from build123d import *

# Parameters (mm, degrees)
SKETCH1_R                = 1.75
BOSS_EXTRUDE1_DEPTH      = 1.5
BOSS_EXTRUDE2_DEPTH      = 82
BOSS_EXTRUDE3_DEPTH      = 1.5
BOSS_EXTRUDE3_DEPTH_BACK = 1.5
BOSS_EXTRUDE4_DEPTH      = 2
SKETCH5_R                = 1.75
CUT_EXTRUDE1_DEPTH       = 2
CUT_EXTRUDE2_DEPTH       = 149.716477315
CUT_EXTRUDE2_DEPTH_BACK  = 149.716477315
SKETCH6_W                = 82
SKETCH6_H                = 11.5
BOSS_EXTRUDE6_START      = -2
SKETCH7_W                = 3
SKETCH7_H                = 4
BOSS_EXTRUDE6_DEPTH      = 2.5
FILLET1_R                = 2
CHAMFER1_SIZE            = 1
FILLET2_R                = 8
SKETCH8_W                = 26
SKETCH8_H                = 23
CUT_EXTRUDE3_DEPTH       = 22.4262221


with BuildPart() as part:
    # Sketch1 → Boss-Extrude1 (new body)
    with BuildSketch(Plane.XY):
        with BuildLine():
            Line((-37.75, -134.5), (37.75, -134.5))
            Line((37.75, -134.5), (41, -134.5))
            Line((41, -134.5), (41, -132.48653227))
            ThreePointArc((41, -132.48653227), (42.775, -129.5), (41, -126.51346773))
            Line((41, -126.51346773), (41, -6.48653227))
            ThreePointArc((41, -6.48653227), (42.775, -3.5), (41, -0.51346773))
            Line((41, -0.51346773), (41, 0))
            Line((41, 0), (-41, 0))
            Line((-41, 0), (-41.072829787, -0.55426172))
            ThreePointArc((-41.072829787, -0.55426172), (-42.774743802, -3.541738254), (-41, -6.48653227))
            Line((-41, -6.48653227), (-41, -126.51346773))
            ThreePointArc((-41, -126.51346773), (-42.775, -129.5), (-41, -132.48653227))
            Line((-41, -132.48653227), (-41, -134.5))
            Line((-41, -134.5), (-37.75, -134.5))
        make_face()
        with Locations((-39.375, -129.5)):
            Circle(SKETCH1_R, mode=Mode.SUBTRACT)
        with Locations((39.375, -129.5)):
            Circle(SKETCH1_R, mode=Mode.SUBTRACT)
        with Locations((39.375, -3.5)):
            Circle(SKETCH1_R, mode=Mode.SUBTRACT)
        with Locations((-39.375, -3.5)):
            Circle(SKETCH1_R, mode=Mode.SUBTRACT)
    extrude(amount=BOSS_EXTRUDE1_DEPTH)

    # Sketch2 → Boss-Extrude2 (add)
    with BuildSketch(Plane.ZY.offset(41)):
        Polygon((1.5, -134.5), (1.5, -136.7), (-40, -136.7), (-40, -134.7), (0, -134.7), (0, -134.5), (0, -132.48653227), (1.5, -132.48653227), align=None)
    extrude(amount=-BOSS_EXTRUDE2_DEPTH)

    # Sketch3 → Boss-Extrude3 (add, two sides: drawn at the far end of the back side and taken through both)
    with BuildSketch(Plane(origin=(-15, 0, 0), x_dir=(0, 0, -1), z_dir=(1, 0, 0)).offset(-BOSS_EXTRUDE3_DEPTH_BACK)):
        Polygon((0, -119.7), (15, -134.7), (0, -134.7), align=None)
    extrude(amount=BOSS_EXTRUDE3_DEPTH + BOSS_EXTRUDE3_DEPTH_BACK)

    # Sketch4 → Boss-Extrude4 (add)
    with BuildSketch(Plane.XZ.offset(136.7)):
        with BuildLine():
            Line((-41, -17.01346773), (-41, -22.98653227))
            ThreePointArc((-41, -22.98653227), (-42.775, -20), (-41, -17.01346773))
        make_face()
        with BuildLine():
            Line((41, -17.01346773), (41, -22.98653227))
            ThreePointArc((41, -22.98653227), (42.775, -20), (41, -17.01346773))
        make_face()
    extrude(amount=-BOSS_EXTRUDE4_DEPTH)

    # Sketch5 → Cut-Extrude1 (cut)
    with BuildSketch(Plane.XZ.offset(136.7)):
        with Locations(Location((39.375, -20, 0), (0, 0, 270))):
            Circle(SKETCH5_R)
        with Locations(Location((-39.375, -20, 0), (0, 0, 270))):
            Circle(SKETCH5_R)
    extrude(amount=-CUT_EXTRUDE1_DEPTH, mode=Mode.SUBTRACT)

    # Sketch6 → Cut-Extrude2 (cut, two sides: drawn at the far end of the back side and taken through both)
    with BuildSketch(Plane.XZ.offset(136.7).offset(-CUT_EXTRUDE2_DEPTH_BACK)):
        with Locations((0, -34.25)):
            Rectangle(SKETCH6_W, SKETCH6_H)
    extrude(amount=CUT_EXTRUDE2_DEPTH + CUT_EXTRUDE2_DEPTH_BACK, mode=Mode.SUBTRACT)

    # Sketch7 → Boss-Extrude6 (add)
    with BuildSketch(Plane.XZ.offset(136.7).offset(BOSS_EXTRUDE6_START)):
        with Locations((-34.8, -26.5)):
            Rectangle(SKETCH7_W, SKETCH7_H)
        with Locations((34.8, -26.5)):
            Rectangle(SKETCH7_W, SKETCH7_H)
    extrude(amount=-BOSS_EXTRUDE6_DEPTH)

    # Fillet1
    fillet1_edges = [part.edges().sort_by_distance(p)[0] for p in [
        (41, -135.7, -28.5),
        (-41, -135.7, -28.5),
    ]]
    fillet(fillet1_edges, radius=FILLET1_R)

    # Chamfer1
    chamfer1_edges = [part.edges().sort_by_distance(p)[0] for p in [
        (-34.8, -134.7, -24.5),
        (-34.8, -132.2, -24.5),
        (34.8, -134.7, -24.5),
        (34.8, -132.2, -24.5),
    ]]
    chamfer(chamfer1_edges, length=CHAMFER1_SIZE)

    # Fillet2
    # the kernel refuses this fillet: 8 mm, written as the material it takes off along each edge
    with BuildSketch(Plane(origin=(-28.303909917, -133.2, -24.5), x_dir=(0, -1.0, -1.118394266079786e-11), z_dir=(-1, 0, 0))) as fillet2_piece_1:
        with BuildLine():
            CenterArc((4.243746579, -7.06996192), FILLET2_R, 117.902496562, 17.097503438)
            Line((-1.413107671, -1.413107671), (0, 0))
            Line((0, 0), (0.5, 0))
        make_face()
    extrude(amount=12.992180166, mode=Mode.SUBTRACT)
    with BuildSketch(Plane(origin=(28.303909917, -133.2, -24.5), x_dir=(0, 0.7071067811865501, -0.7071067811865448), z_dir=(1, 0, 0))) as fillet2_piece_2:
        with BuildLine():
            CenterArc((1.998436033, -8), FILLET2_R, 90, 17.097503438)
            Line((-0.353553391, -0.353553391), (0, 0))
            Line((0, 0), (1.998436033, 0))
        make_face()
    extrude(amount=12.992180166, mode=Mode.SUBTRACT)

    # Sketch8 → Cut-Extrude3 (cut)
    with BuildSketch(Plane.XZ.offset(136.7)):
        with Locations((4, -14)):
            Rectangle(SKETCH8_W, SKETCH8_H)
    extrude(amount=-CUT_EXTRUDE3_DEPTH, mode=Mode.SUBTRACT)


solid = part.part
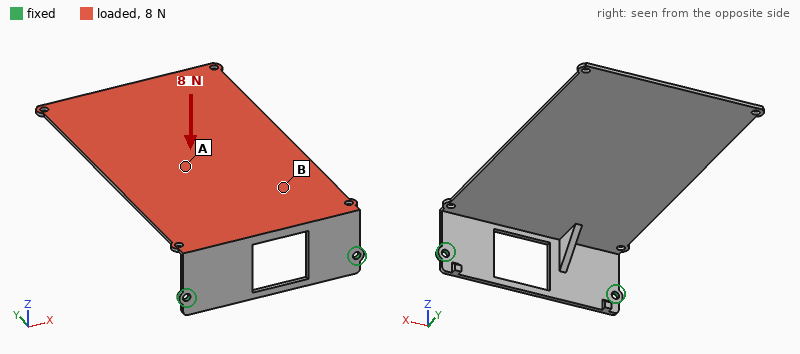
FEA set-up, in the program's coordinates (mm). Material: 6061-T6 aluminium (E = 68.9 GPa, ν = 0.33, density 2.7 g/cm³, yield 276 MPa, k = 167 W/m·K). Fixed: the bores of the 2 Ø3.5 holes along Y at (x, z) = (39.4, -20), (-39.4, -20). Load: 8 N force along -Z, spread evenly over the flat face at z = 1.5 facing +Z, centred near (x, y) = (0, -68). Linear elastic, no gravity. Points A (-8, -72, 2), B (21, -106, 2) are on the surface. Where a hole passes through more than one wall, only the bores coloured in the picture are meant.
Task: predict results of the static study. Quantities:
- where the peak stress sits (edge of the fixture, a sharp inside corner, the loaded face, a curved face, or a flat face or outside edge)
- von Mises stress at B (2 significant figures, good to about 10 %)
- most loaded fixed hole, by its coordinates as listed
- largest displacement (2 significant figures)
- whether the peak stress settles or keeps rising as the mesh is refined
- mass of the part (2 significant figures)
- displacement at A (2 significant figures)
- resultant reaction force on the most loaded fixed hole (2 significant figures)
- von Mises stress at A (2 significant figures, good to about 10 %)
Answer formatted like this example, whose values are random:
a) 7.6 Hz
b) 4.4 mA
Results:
a) edge of the fixture
b) 8.8 MPa
c) (-39.4, -20)
d) 1.8 mm
e) keeps rising
f) 56 g
g) 0.61 mm
h) 6.0 N
i) 4.4 MPa
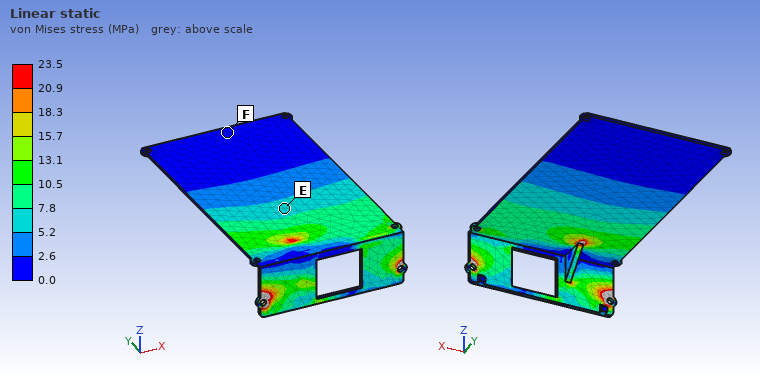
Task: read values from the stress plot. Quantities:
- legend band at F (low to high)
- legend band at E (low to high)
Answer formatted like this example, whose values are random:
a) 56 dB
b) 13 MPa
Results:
a) 0.0 to 2.6 MPa
b) 5.2 to 7.8 MPa
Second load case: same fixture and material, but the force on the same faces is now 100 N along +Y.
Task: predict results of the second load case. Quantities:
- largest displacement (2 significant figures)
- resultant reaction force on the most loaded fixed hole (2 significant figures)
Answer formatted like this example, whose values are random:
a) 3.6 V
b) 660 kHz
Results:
a) 1.7 mm
b) 51 N
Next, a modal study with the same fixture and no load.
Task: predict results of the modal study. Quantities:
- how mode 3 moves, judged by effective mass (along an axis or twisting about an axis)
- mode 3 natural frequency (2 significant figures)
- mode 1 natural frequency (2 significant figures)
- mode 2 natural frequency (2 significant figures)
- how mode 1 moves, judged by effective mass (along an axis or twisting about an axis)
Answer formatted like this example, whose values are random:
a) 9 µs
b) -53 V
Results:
a) along X
b) 320 Hz
c) 63 Hz
d) 230 Hz
e) along Z
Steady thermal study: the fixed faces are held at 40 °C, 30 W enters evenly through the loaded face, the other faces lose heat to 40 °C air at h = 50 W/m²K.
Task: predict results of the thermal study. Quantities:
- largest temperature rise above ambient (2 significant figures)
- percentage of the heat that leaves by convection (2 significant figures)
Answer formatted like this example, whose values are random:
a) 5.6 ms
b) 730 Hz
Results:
a) 41 K
b) 72 %
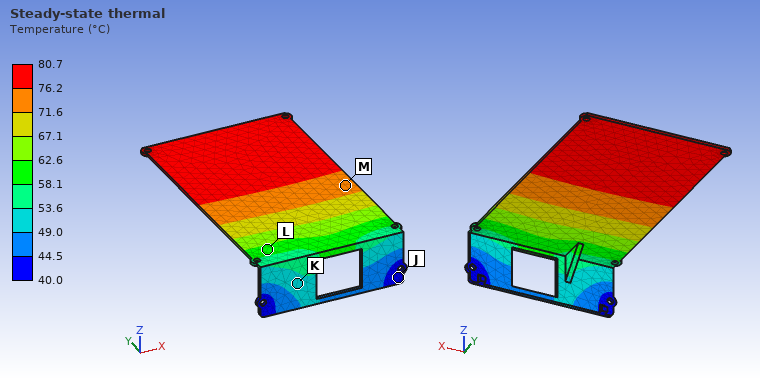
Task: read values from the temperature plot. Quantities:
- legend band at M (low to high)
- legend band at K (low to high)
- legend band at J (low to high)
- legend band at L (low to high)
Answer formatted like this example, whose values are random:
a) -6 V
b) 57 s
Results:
a) 71.6 to 76.2 °C
b) 49.0 to 53.6 °C
c) 40.0 to 44.5 °C
d) 58.1 to 62.6 °C
